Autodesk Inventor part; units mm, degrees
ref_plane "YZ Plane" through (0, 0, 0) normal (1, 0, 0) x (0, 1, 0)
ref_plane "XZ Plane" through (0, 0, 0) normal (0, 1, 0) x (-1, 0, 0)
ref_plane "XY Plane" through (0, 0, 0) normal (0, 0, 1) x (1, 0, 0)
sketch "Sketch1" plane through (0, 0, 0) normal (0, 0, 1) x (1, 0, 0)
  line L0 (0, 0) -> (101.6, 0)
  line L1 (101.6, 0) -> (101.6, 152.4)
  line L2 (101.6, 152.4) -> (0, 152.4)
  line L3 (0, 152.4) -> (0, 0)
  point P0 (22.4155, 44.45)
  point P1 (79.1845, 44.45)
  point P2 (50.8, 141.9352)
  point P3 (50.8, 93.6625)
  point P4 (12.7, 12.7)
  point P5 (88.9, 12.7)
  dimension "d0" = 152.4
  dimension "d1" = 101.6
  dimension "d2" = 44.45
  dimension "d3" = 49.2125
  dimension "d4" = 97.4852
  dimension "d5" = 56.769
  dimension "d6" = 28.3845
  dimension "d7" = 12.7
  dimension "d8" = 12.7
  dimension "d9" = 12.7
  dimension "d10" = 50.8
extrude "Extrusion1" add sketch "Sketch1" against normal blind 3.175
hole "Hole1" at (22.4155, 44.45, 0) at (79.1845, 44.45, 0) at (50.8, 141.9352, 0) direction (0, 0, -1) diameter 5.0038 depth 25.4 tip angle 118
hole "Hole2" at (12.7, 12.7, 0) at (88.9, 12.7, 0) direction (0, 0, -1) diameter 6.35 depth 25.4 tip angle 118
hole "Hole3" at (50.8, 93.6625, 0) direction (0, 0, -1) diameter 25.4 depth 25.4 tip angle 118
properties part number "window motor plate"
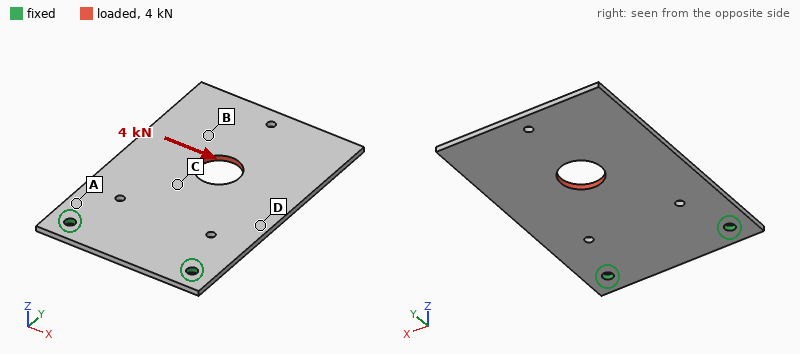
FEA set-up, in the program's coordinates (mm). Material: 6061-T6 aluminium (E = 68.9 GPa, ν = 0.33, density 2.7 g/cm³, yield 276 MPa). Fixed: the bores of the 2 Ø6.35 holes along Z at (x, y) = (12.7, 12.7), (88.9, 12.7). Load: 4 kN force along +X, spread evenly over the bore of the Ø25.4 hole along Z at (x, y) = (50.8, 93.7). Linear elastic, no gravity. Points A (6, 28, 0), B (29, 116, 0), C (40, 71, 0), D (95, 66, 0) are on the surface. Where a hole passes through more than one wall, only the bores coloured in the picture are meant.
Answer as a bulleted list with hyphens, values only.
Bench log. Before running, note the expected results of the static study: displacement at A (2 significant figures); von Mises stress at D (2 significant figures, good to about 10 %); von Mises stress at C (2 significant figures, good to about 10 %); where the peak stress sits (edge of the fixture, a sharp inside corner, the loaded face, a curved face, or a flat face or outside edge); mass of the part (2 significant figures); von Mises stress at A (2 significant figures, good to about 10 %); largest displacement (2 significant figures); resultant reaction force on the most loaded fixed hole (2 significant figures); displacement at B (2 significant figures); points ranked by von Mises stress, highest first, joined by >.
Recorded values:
- 0.024 mm
- 21 MPa
- 31 MPa
- edge of the fixture
- 130 g
- 43 MPa
- 0.16 mm
- 4.6 kN
- 0.12 mm
- A > C > D > B
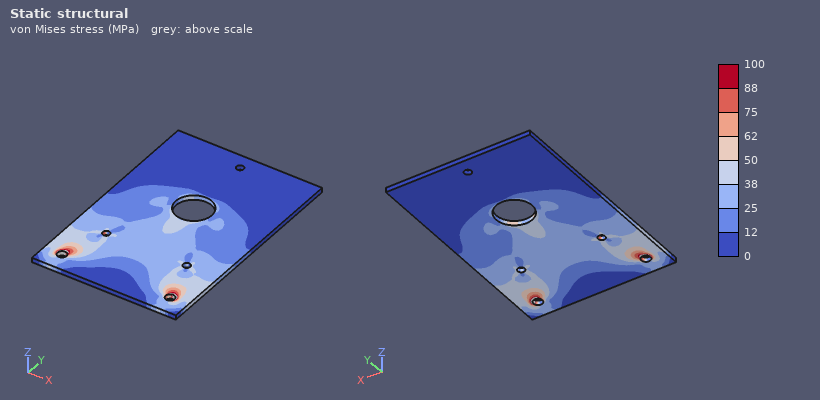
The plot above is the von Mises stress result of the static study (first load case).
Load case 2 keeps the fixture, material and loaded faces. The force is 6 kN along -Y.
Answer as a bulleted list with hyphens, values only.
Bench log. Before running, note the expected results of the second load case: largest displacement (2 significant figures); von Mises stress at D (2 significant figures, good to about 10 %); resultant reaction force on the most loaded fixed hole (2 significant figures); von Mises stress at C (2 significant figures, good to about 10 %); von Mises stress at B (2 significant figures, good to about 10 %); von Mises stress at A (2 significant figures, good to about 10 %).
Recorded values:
- 42 µm
- 16 MPa
- 3.1 kN
- 24 MPa
- 12 MPa
- 28 MPa
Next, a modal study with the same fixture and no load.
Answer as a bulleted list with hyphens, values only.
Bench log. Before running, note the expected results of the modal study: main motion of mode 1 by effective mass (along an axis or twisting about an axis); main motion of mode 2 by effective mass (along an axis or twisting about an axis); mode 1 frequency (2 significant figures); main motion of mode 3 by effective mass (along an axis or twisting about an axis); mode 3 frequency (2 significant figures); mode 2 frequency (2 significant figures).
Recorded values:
- along Z
- twisting about Y
- 130 Hz
- along Z
- 780 Hz
- 410 Hz
